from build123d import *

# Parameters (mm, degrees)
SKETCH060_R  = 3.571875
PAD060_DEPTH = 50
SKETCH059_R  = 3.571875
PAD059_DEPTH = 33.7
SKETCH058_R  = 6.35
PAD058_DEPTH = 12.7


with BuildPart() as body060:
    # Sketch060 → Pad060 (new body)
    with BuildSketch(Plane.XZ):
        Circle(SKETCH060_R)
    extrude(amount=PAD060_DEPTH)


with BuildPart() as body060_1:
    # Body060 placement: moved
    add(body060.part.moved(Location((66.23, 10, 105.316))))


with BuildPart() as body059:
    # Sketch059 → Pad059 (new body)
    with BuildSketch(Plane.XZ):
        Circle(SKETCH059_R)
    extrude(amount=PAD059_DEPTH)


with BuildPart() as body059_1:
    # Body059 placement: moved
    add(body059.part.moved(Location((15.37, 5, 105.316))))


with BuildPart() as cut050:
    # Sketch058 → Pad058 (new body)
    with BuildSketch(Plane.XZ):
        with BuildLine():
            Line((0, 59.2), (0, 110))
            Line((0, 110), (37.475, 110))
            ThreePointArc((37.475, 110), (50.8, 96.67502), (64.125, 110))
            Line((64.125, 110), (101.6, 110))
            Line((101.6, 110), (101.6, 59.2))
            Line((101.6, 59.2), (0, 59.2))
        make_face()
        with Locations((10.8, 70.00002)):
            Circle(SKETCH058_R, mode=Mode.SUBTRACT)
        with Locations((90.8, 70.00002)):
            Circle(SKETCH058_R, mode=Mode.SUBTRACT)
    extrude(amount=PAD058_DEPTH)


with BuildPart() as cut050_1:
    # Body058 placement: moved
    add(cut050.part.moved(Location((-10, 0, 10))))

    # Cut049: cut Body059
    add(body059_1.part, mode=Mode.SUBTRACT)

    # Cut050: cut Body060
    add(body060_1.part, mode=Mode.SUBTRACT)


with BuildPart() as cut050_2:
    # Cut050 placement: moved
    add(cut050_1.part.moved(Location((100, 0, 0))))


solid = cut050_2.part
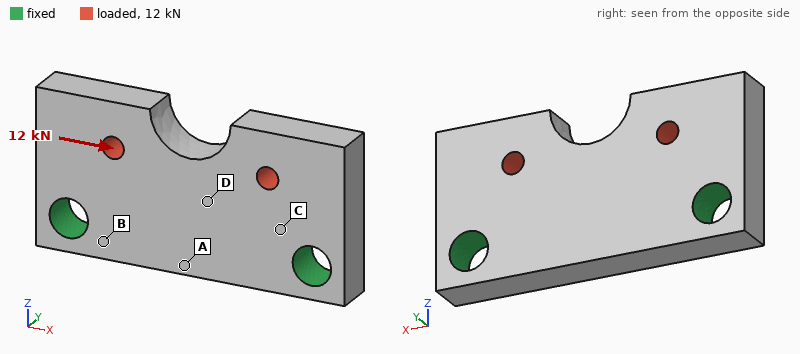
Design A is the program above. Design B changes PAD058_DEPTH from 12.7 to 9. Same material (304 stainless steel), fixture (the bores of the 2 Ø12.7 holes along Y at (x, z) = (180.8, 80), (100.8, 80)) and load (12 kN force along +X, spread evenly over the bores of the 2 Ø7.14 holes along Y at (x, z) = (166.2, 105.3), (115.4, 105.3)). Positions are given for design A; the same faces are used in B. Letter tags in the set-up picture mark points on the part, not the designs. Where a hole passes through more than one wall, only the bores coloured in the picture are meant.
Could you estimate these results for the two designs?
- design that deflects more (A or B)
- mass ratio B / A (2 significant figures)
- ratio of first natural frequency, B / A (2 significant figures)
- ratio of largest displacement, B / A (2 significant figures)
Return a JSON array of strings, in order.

["B", "0.71", "0.77", "1.4"]
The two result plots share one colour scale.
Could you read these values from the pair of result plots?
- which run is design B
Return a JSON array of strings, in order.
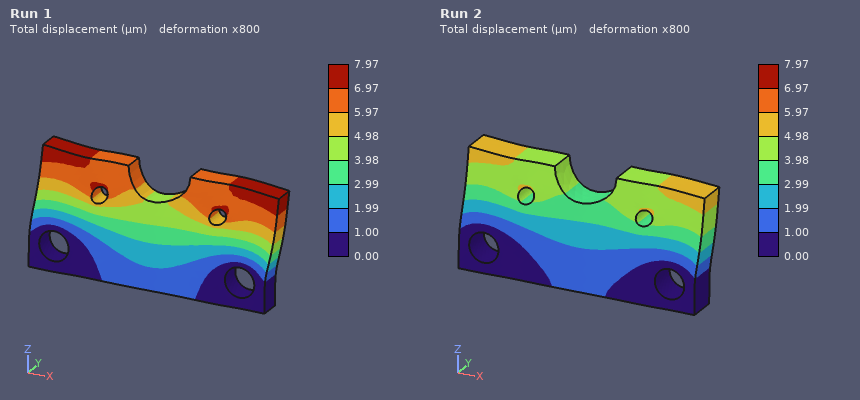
["Run 1"]
